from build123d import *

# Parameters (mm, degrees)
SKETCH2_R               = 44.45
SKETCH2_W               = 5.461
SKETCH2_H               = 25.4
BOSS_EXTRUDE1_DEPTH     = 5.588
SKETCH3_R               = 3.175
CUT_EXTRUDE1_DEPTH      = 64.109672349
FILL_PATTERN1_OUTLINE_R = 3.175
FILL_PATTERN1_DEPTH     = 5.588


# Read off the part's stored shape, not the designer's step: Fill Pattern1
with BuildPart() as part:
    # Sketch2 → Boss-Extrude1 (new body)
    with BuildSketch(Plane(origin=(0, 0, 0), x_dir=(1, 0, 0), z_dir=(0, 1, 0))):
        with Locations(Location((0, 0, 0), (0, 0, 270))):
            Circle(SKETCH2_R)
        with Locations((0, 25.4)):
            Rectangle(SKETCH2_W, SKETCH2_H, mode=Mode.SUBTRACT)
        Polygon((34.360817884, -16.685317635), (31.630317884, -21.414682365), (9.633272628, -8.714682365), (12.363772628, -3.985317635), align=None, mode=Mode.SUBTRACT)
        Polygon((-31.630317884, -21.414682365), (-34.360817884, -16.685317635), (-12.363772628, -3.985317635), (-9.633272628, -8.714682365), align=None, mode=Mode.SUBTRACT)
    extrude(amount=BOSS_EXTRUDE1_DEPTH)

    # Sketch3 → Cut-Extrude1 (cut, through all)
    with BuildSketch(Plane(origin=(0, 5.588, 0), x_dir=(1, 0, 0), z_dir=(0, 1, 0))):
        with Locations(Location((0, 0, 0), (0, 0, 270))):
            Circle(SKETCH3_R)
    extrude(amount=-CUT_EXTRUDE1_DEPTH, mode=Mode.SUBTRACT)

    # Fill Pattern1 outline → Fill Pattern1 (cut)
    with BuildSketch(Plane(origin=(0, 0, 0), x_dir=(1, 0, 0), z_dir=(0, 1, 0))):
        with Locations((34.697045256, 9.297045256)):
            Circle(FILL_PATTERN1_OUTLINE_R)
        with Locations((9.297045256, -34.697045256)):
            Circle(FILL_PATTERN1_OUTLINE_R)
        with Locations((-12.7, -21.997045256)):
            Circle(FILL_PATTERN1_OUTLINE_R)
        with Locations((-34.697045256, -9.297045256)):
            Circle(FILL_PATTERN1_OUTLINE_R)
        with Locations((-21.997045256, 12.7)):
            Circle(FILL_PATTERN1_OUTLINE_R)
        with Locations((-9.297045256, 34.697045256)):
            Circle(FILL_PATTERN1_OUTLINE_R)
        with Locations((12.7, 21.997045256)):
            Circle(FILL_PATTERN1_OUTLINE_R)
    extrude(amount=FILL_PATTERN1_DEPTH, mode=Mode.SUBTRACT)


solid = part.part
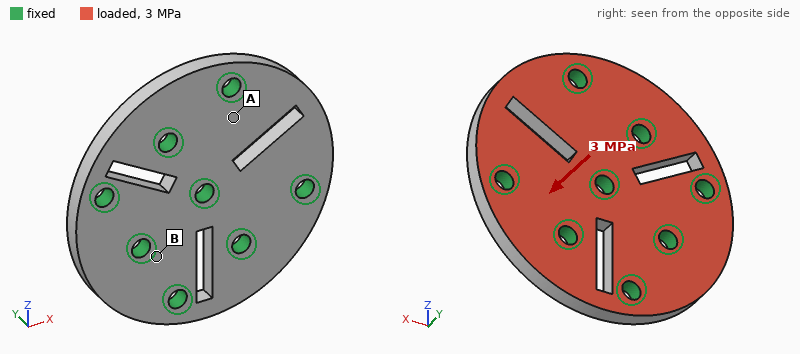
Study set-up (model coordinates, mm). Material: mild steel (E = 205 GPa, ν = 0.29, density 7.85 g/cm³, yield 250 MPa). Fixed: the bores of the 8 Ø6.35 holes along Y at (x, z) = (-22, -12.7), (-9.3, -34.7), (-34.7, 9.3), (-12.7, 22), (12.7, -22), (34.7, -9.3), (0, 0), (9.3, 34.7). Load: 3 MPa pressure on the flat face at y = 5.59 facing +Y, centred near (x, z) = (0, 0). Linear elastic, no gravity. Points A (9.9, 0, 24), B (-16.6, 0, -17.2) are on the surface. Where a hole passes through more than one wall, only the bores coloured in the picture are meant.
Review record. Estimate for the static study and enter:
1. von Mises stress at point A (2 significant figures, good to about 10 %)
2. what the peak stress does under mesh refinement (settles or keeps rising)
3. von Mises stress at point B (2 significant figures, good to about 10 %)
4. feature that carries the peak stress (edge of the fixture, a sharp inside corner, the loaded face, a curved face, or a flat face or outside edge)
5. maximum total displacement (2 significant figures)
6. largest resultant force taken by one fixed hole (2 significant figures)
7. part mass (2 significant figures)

46 MPa
keeps rising
19 MPa
edge of the fixture
37 µm
2.6 kN
240 g
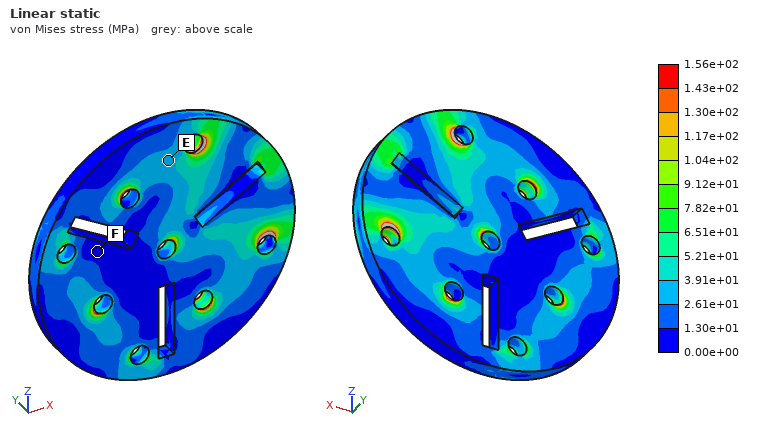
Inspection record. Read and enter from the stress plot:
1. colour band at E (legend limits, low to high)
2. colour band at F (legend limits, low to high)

2.61e+01 to 3.91e+01 MPa
0.00e+00 to 1.30e+01 MPa
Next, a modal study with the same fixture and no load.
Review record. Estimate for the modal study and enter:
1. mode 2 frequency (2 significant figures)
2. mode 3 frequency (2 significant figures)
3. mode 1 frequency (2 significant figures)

15 kHz
15 kHz
9100 Hz
